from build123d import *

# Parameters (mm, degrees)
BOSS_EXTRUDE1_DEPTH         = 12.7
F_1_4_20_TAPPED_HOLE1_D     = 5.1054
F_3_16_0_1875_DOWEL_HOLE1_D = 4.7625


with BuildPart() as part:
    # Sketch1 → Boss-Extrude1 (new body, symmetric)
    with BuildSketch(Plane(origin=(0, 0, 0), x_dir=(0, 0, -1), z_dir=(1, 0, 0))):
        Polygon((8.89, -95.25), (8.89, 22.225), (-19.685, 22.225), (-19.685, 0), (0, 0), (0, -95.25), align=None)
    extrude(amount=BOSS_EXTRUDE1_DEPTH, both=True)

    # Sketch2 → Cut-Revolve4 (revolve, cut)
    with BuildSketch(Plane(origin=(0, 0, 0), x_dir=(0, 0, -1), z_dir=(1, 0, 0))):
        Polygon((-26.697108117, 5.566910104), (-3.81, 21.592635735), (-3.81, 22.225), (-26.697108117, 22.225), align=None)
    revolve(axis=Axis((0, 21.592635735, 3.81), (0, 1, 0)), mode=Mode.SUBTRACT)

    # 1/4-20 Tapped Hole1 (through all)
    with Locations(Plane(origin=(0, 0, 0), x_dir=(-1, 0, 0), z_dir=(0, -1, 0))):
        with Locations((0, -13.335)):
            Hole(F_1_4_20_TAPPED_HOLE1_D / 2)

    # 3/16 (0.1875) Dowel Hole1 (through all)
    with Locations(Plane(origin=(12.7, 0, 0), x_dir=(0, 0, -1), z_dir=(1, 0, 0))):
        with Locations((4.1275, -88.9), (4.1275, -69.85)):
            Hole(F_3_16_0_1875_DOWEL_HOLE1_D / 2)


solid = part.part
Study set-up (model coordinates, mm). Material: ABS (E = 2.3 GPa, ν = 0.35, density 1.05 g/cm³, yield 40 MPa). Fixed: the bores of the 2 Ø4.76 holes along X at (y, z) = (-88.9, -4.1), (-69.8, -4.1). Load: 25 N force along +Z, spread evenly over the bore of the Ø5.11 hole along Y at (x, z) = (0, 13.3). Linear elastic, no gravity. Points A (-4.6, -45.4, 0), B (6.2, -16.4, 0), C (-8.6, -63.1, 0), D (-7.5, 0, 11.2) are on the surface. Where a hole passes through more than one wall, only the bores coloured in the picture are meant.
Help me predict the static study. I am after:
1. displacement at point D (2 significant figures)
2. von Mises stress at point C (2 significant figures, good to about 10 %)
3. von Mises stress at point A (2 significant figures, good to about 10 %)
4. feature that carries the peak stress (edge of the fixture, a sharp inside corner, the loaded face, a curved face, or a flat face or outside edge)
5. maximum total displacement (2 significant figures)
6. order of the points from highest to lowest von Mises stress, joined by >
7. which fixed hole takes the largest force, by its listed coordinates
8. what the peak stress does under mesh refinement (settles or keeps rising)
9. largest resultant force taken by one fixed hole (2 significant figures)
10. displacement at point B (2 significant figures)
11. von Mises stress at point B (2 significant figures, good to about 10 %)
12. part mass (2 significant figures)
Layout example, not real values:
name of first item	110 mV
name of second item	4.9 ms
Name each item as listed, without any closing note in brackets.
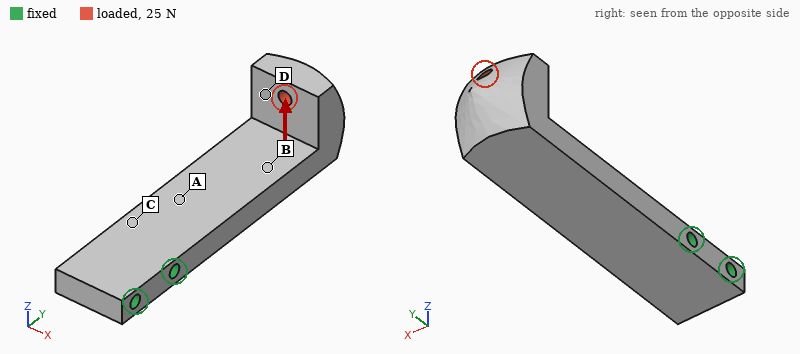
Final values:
displacement at point D	1.0 mm
von Mises stress at point C	5.1 MPa
von Mises stress at point A	3.9 MPa
feature that carries the peak stress	edge of the fixture
maximum total displacement	1.4 mm
order of the points from highest to lowest von Mises stress, joined by >	C > A > B > D
which fixed hole takes the largest force, by its listed coordinates	(-69.8, -4.1)
what the peak stress does under mesh refinement	keeps rising
largest resultant force taken by one fixed hole	42 N
displacement at point B	0.63 mm
von Mises stress at point B	1.8 MPa
part mass	32 g
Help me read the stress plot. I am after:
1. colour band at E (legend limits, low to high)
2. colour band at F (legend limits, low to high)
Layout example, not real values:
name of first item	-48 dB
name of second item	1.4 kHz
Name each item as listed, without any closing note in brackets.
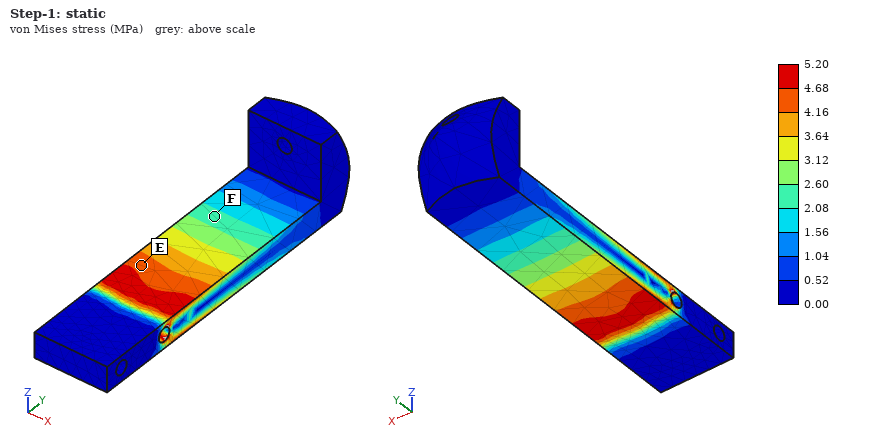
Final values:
colour band at E	4.16 to 4.68 MPa
colour band at F	2.08 to 2.60 MPa
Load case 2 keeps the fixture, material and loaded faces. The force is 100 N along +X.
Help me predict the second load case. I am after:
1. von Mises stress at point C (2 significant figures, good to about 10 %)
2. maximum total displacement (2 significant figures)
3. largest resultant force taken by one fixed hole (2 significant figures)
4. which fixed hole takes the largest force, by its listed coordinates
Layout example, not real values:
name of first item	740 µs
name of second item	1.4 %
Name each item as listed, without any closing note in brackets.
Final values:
von Mises stress at point C	5.2 MPa
maximum total displacement	1.3 mm
largest resultant force taken by one fixed hole	110 N
which fixed hole takes the largest force, by its listed coordinates	(-69.8, -4.1)
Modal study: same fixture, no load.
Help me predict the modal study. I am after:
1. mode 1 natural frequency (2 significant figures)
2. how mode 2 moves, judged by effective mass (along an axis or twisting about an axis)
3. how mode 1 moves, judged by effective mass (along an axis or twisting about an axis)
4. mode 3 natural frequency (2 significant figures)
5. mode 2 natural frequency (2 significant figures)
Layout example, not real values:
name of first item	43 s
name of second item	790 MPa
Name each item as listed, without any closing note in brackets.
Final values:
mode 1 natural frequency	200 Hz
how mode 2 moves, judged by effective mass	along X
how mode 1 moves, judged by effective mass	along Z
mode 3 natural frequency	1000 Hz
mode 2 natural frequency	520 Hz
